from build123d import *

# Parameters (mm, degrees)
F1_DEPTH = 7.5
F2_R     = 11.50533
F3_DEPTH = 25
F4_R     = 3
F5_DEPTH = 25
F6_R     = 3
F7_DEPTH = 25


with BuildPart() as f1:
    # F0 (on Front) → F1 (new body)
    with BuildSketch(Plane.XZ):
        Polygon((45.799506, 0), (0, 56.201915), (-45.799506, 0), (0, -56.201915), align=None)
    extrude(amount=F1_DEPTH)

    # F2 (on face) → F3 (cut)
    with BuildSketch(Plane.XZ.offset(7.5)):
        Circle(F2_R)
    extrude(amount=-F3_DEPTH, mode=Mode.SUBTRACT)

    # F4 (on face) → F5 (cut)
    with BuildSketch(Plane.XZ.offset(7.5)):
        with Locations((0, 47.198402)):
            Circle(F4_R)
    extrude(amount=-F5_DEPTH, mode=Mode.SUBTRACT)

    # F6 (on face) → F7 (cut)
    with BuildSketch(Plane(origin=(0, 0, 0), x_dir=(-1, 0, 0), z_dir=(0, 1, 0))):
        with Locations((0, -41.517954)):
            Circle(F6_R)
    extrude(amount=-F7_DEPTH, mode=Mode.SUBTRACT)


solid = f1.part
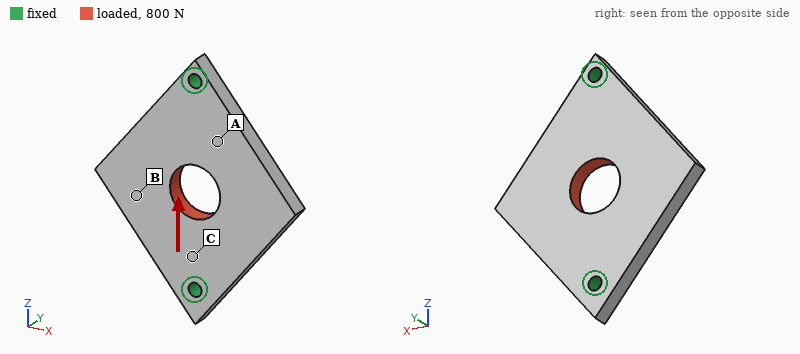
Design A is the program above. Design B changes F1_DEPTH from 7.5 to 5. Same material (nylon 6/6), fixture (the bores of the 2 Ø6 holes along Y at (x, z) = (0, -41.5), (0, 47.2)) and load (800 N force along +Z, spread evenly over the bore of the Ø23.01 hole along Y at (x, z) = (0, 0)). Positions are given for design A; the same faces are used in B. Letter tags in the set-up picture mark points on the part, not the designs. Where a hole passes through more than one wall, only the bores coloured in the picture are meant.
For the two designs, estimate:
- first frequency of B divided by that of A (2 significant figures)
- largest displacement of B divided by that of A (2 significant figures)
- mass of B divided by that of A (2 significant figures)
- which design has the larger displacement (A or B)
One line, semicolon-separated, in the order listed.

0.70; 1.5; 0.67; B
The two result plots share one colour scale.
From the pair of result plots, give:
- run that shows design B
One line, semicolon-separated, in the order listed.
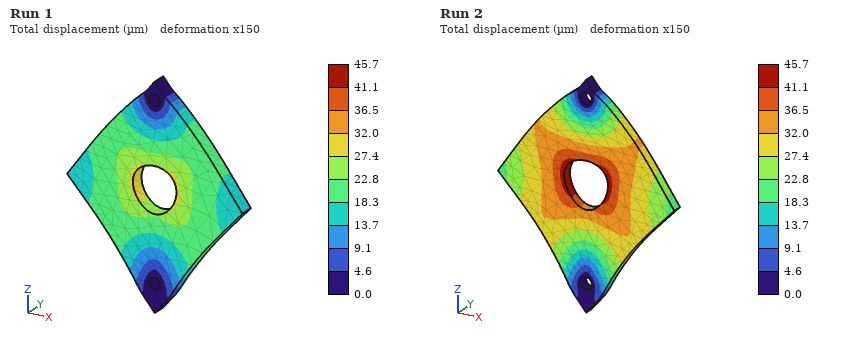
Run 2
